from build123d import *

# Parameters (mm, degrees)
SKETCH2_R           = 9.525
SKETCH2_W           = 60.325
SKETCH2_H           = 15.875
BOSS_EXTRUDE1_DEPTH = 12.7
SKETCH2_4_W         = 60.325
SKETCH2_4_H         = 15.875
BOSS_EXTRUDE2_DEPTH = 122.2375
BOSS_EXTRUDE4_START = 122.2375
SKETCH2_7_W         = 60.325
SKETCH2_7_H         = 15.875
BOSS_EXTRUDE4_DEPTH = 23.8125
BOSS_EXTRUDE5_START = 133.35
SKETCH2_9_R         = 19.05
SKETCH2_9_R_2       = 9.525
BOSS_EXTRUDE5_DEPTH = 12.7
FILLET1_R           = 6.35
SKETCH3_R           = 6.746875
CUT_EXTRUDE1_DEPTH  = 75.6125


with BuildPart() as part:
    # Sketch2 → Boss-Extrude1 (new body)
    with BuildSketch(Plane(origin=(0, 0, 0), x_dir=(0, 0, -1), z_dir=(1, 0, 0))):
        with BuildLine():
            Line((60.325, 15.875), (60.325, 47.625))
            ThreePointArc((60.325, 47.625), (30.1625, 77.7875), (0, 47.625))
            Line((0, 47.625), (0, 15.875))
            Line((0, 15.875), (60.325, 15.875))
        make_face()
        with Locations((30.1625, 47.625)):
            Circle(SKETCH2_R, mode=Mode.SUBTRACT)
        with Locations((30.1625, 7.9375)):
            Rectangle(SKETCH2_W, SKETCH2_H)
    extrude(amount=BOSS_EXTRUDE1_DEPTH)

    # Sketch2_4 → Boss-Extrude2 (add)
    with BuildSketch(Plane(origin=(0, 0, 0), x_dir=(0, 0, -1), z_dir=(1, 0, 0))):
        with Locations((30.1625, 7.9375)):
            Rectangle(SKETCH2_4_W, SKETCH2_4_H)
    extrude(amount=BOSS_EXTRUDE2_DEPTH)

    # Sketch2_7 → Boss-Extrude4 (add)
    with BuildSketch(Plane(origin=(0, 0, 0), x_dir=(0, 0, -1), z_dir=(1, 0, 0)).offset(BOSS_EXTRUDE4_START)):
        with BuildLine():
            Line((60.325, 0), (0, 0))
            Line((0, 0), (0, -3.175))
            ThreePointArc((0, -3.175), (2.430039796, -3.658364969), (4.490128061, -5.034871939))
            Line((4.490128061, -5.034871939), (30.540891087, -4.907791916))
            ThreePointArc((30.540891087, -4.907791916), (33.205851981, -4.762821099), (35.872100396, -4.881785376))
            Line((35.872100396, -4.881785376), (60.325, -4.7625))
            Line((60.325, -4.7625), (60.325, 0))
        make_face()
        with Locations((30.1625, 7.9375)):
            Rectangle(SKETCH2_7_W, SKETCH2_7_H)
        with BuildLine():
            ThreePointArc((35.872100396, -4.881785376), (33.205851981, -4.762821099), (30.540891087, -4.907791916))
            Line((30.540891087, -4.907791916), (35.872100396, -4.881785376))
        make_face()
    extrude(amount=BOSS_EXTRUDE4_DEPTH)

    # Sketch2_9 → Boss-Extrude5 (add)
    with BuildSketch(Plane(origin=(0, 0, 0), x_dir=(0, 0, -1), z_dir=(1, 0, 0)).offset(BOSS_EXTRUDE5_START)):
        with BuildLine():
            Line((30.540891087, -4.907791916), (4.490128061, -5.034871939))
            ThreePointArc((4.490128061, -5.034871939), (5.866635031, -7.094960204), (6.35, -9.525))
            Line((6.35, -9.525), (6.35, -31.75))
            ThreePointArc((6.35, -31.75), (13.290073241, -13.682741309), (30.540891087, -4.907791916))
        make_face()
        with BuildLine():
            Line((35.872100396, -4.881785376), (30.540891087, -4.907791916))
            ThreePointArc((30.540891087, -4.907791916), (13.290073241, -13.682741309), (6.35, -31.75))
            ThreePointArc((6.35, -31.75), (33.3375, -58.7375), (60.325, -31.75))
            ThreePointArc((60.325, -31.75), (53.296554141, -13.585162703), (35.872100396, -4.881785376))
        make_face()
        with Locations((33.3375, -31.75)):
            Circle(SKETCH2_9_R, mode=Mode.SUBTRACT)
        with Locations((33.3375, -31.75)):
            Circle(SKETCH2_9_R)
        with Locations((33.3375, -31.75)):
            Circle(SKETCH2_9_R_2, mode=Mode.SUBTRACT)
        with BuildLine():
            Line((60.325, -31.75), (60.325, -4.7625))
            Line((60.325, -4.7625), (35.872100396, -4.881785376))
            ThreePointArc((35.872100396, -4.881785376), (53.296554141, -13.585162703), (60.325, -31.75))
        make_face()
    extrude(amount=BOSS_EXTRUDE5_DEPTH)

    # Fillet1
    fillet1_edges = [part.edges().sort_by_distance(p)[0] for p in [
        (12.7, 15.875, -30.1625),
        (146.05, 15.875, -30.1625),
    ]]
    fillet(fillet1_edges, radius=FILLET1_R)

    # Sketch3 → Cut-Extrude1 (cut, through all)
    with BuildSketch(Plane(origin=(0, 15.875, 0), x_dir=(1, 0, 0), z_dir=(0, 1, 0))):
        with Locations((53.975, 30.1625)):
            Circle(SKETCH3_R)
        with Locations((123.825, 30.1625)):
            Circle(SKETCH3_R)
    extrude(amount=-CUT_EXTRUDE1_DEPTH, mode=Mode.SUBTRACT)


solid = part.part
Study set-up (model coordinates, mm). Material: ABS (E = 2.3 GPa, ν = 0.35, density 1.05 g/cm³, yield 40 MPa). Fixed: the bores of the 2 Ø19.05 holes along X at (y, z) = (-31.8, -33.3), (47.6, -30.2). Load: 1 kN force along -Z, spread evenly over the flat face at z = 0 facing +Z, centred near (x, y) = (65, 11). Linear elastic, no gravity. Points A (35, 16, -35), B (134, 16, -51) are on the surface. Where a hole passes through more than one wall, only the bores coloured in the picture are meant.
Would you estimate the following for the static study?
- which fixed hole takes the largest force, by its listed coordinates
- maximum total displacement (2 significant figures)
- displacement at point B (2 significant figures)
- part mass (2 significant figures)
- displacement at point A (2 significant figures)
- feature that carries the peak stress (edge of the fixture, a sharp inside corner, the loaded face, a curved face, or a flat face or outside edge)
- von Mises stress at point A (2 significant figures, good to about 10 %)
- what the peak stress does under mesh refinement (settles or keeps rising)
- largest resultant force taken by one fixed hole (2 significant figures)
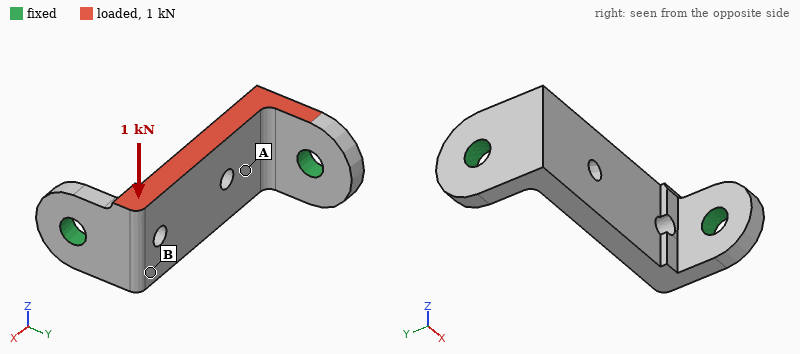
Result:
(47.6, -30.2)
0.13 mm
0.093 mm
220 g
0.094 mm
edge of the fixture
1.2 MPa
keeps rising
560 N
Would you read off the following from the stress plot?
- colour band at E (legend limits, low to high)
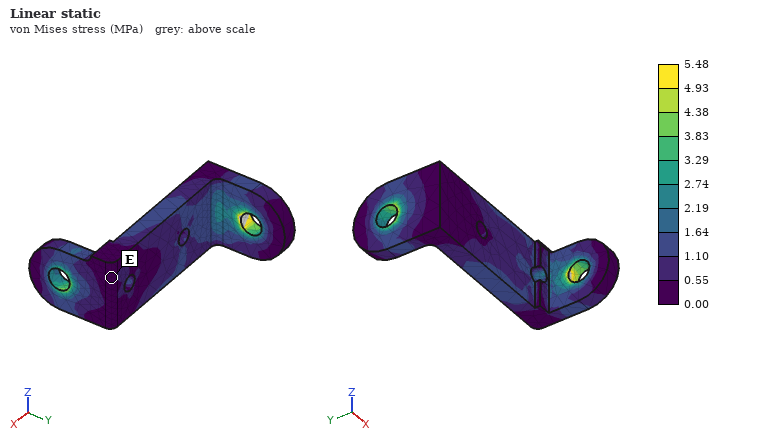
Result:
0.00 to 0.55 MPa
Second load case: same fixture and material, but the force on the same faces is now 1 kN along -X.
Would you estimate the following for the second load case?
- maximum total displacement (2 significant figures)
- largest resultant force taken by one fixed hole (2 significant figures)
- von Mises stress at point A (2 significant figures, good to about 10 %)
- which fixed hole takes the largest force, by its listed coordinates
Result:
0.34 mm
580 N
1.6 MPa
(47.6, -30.2)
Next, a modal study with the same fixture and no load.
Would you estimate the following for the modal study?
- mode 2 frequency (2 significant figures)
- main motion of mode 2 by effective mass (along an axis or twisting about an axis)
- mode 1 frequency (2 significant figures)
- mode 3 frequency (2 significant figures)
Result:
1200 Hz
along Z
640 Hz
1400 Hz
